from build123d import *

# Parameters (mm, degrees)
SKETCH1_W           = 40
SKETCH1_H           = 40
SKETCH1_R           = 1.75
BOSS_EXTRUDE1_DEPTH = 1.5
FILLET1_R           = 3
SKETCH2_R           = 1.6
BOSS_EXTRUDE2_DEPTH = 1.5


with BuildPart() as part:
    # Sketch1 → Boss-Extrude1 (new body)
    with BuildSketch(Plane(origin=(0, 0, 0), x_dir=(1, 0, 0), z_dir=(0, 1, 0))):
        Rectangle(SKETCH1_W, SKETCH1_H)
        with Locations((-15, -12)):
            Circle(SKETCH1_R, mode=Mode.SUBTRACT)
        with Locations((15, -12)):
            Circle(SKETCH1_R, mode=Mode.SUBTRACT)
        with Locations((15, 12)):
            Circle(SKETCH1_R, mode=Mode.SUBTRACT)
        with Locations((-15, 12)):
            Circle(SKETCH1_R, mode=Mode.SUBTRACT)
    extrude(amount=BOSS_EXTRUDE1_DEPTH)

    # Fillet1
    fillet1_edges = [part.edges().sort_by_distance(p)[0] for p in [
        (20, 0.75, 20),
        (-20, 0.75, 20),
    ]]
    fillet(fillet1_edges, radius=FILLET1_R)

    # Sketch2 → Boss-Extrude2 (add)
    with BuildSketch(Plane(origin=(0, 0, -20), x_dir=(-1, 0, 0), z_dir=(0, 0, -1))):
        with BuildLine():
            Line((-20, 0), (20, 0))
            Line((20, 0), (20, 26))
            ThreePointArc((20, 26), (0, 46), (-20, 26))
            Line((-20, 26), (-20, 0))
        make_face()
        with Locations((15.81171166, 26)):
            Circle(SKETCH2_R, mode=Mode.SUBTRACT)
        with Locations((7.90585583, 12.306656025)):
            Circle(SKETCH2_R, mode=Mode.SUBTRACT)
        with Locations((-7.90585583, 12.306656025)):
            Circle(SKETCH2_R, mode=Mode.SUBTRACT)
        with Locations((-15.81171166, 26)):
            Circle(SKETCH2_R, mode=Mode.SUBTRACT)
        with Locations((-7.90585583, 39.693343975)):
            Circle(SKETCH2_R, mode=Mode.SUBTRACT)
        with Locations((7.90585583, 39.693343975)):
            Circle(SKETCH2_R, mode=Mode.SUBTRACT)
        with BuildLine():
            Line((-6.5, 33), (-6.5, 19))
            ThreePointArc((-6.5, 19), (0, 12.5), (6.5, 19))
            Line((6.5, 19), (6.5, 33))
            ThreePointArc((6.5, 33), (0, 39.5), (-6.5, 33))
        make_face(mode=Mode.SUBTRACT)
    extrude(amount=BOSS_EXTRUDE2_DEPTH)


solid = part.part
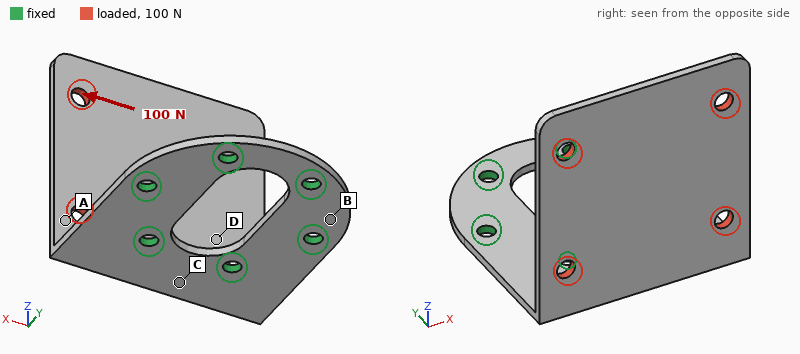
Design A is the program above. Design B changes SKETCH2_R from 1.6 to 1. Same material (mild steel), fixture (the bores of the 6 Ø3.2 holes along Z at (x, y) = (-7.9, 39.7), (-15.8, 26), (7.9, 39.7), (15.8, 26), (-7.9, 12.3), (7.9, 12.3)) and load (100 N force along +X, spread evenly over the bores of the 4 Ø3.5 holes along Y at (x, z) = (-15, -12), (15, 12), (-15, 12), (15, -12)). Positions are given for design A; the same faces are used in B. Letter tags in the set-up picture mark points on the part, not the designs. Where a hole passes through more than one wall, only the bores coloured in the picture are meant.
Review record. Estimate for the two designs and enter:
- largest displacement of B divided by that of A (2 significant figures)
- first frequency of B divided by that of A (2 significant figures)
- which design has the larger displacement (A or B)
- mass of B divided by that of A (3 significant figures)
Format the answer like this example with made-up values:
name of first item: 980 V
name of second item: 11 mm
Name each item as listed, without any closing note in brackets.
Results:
largest displacement of B divided by that of A: 1.2
first frequency of B divided by that of A: 0.98
which design has the larger displacement: B
mass of B divided by that of A: 1.01
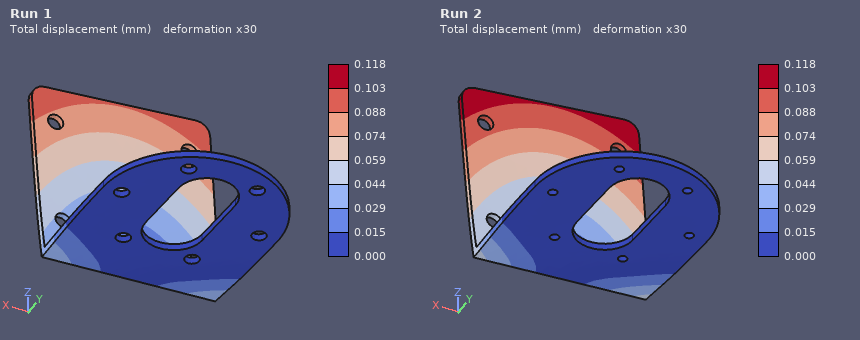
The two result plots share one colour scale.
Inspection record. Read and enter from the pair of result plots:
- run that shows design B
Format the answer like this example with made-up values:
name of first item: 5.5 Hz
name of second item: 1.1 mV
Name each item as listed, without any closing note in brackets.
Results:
run that shows design B: Run 2
